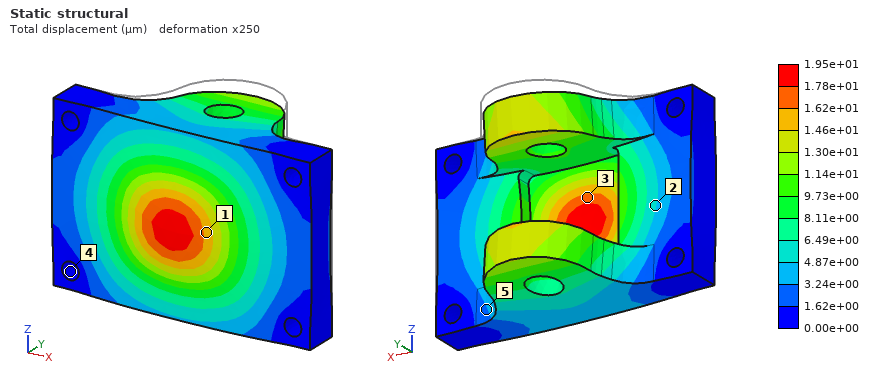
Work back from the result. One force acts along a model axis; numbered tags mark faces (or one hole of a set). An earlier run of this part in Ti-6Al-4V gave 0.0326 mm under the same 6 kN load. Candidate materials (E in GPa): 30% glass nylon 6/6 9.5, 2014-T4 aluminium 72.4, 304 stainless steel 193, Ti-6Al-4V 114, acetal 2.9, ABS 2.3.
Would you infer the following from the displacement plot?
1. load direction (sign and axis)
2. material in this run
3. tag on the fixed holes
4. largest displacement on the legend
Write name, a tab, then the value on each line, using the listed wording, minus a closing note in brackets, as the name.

load direction	-Y
material in this run	304 stainless steel
tag on the fixed holes	4
largest displacement on the legend	1.95e+01 µm
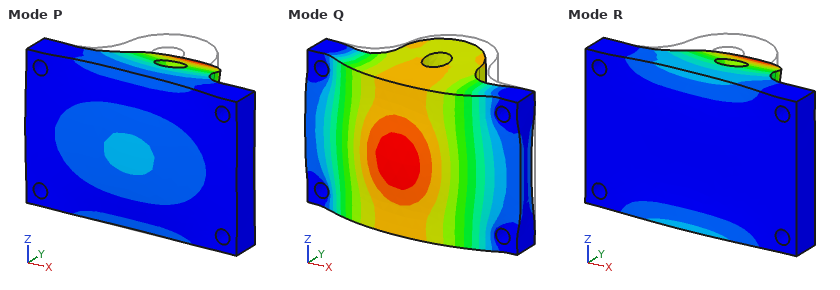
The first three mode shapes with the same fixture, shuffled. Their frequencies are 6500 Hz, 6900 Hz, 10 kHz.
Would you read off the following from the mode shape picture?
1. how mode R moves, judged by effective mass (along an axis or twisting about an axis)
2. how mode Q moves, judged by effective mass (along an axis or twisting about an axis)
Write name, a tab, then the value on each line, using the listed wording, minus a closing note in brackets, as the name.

how mode R moves, judged by effective mass	along Z
how mode Q moves, judged by effective mass	along Y
